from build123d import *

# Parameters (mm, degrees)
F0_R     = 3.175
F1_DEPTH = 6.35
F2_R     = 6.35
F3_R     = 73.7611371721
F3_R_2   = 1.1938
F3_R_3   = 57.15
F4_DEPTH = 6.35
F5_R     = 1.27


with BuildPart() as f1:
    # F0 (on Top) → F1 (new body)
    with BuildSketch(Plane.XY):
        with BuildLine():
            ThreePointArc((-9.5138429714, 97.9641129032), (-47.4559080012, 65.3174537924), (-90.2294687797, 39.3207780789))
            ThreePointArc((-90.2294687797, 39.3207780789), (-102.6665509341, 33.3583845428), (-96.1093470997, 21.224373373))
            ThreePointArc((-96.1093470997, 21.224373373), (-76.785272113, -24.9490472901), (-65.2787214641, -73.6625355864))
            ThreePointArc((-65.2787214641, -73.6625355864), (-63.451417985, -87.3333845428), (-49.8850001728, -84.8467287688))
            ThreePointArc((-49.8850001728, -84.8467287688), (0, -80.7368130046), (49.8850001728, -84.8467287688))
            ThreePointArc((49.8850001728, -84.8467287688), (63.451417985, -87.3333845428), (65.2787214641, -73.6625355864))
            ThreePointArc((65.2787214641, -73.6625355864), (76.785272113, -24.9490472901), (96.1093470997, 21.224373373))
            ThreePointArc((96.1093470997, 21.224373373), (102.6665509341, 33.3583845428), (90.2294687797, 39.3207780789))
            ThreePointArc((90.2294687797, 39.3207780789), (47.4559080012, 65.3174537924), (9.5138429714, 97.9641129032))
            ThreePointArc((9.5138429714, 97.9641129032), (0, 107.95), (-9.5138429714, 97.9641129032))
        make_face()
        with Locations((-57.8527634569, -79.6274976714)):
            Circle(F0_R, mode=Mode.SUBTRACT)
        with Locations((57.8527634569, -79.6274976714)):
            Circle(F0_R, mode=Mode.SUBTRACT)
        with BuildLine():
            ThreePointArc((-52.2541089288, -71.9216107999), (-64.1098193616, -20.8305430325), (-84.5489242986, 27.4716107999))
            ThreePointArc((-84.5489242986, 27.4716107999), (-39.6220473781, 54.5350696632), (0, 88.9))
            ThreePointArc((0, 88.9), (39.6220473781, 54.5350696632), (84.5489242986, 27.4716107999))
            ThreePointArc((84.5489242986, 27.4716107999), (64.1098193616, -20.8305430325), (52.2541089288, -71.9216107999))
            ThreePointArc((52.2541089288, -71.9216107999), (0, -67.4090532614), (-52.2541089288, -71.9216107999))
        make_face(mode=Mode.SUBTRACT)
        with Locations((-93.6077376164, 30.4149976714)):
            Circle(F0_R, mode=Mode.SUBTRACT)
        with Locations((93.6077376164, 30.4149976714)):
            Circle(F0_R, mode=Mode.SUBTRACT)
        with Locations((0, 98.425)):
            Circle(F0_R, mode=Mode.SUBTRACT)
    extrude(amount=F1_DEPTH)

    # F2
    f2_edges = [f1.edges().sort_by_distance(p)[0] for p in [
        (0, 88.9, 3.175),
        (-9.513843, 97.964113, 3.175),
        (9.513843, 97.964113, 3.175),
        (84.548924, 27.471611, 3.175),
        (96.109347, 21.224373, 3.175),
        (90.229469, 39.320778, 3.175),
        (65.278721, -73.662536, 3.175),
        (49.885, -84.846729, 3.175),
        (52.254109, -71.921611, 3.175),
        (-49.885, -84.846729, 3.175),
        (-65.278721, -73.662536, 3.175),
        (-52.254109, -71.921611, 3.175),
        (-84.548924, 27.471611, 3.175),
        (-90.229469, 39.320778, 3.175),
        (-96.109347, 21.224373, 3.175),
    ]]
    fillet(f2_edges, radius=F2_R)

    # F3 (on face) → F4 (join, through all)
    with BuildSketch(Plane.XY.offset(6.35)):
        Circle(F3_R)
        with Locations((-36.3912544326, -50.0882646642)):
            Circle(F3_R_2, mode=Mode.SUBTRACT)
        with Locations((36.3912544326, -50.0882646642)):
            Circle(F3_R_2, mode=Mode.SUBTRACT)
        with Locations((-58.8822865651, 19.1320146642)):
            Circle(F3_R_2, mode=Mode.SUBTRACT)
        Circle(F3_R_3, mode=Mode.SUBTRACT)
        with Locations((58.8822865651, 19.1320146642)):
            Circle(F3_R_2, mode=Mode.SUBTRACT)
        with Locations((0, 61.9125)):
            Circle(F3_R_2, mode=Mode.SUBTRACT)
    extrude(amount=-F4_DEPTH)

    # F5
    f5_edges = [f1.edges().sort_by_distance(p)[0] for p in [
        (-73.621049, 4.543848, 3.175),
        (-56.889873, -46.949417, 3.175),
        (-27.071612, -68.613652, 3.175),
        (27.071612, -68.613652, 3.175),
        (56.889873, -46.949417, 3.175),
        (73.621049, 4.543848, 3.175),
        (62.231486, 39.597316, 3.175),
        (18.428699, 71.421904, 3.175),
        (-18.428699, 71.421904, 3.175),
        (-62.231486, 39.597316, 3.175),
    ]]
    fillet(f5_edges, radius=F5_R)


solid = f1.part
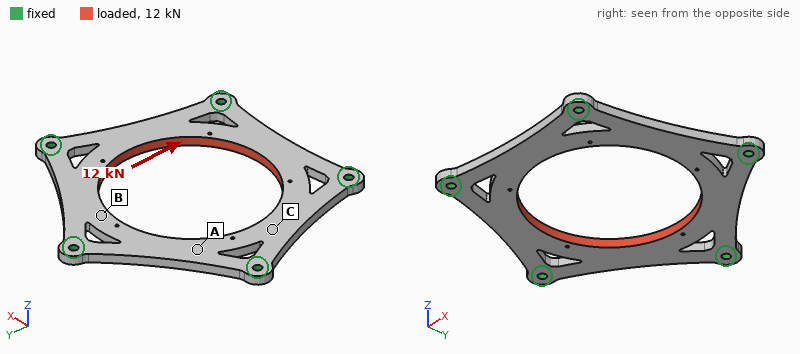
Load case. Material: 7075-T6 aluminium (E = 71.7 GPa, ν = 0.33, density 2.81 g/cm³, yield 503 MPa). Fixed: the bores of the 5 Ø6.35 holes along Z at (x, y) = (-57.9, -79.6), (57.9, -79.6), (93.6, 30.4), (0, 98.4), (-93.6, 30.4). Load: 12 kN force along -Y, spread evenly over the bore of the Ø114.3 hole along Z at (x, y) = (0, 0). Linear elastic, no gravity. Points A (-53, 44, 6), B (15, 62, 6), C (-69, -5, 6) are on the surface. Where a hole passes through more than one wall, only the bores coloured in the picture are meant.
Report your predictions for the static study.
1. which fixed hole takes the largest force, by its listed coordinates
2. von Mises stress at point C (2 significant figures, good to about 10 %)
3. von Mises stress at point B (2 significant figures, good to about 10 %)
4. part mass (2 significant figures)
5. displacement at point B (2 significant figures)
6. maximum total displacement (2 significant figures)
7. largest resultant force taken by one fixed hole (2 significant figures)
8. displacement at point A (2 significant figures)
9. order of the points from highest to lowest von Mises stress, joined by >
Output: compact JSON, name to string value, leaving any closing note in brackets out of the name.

{"which fixed hole takes the largest force, by its listed coordinates": "(0, 98.4)", "von Mises stress at point C": "11 MPa", "von Mises stress at point B": "17 MPa", "part mass": "240 g", "displacement at point B": "20 µm", "maximum total displacement": "28 µm", "largest resultant force taken by one fixed hole": "3.2 kN", "displacement at point A": "23 µm", "order of the points from highest to lowest von Mises stress, joined by >": "B > C > A"}
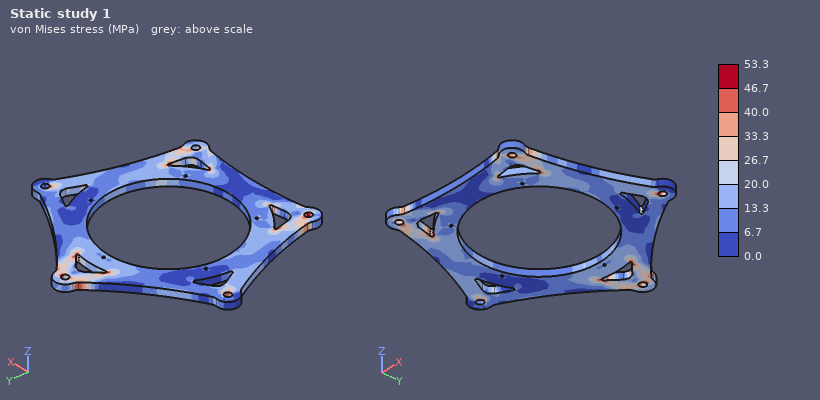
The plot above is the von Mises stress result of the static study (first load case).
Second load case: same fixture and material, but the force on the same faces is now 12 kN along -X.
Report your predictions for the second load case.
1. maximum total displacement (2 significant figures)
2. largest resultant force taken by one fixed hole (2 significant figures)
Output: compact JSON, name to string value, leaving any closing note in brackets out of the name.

{"maximum total displacement": "27 µm", "largest resultant force taken by one fixed hole": "3.1 kN"}
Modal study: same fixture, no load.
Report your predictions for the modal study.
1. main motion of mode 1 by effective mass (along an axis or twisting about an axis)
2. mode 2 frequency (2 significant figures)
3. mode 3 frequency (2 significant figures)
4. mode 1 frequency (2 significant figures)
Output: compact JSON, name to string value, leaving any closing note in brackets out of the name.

{"main motion of mode 1 by effective mass": "along Z", "mode 2 frequency": "2100 Hz", "mode 3 frequency": "2100 Hz", "mode 1 frequency": "1700 Hz"}
